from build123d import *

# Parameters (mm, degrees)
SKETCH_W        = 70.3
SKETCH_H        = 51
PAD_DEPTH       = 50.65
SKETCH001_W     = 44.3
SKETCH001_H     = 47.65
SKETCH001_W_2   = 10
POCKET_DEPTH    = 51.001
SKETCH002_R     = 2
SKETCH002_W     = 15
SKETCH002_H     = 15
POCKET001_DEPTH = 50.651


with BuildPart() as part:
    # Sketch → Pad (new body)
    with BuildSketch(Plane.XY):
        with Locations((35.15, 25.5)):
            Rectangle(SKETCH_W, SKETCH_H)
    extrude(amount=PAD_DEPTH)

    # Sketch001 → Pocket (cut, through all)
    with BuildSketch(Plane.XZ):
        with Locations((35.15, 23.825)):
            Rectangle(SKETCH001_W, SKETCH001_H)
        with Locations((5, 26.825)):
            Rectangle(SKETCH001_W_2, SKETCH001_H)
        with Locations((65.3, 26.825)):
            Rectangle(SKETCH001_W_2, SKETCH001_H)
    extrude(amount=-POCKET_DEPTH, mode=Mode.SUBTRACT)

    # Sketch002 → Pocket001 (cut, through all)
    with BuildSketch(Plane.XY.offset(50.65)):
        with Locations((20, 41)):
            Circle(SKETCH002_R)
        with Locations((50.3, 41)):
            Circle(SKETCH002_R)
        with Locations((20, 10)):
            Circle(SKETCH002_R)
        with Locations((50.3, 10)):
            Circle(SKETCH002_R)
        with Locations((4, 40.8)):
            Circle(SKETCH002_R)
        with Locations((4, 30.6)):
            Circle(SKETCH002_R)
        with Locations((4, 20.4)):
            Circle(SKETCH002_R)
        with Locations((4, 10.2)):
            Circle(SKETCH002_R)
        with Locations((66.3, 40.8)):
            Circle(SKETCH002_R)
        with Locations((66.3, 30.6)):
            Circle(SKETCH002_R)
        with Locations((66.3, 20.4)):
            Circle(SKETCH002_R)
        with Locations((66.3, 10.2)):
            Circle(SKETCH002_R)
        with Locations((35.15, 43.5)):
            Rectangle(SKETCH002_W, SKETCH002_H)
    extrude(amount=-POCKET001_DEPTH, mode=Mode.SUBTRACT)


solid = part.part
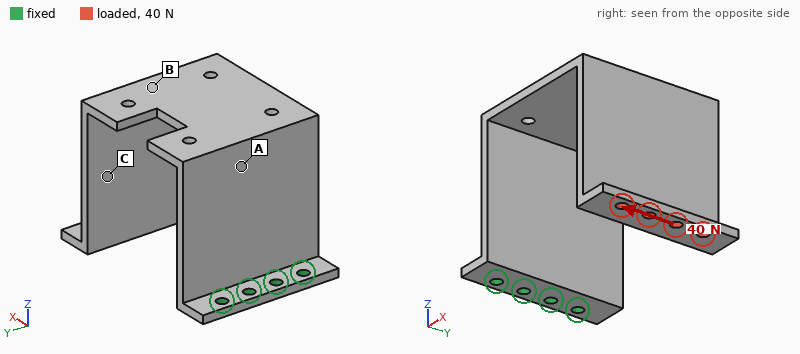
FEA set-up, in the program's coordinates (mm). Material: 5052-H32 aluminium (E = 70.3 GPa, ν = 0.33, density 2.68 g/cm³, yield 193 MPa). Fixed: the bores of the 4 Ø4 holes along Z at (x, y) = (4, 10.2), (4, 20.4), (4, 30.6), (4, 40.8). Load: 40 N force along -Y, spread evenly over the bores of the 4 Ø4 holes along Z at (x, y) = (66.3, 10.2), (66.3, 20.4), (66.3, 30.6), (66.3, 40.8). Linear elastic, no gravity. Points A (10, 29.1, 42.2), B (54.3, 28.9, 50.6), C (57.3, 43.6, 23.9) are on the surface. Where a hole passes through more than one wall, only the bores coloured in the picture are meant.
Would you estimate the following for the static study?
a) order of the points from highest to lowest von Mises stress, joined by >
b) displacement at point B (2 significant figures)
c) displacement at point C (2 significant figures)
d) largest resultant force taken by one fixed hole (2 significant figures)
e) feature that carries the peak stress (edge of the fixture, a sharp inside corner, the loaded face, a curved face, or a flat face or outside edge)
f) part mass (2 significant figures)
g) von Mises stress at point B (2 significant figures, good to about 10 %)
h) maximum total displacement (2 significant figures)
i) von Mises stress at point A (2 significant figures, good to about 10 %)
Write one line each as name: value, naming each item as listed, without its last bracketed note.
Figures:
order of the points from highest to lowest von Mises stress, joined by >: A > B > C
displacement at point B: 0.29 mm
displacement at point C: 0.59 mm
largest resultant force taken by one fixed hole: 70 N
feature that carries the peak stress: a flat face or outside edge
part mass: 65 g
von Mises stress at point B: 14 MPa
maximum total displacement: 0.92 mm
von Mises stress at point A: 23 MPa
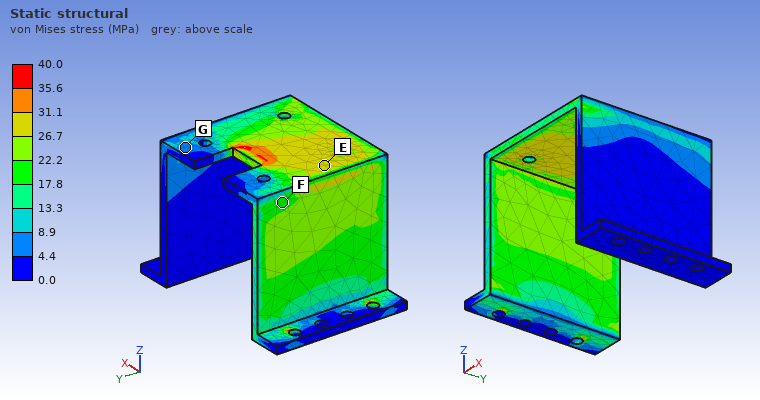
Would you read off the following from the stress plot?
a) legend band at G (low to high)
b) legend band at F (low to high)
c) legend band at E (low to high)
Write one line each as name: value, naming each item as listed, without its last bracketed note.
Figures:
legend band at G: 4.4 to 8.9 MPa
legend band at F: 17.8 to 22.2 MPa
legend band at E: 26.7 to 31.1 MPa
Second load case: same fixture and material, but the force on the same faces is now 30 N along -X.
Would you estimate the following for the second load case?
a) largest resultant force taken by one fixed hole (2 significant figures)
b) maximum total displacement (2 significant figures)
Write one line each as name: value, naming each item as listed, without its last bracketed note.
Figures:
largest resultant force taken by one fixed hole: 13 N
maximum total displacement: 1.0 mm
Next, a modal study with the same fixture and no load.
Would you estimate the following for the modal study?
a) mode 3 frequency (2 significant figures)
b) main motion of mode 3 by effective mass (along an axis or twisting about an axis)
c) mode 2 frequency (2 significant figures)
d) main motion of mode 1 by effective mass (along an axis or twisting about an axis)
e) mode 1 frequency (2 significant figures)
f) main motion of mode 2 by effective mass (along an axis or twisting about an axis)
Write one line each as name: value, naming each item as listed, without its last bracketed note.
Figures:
mode 3 frequency: 350 Hz
main motion of mode 3 by effective mass: along X
mode 2 frequency: 270 Hz
main motion of mode 1 by effective mass: along Z
mode 1 frequency: 180 Hz
main motion of mode 2 by effective mass: along Y
